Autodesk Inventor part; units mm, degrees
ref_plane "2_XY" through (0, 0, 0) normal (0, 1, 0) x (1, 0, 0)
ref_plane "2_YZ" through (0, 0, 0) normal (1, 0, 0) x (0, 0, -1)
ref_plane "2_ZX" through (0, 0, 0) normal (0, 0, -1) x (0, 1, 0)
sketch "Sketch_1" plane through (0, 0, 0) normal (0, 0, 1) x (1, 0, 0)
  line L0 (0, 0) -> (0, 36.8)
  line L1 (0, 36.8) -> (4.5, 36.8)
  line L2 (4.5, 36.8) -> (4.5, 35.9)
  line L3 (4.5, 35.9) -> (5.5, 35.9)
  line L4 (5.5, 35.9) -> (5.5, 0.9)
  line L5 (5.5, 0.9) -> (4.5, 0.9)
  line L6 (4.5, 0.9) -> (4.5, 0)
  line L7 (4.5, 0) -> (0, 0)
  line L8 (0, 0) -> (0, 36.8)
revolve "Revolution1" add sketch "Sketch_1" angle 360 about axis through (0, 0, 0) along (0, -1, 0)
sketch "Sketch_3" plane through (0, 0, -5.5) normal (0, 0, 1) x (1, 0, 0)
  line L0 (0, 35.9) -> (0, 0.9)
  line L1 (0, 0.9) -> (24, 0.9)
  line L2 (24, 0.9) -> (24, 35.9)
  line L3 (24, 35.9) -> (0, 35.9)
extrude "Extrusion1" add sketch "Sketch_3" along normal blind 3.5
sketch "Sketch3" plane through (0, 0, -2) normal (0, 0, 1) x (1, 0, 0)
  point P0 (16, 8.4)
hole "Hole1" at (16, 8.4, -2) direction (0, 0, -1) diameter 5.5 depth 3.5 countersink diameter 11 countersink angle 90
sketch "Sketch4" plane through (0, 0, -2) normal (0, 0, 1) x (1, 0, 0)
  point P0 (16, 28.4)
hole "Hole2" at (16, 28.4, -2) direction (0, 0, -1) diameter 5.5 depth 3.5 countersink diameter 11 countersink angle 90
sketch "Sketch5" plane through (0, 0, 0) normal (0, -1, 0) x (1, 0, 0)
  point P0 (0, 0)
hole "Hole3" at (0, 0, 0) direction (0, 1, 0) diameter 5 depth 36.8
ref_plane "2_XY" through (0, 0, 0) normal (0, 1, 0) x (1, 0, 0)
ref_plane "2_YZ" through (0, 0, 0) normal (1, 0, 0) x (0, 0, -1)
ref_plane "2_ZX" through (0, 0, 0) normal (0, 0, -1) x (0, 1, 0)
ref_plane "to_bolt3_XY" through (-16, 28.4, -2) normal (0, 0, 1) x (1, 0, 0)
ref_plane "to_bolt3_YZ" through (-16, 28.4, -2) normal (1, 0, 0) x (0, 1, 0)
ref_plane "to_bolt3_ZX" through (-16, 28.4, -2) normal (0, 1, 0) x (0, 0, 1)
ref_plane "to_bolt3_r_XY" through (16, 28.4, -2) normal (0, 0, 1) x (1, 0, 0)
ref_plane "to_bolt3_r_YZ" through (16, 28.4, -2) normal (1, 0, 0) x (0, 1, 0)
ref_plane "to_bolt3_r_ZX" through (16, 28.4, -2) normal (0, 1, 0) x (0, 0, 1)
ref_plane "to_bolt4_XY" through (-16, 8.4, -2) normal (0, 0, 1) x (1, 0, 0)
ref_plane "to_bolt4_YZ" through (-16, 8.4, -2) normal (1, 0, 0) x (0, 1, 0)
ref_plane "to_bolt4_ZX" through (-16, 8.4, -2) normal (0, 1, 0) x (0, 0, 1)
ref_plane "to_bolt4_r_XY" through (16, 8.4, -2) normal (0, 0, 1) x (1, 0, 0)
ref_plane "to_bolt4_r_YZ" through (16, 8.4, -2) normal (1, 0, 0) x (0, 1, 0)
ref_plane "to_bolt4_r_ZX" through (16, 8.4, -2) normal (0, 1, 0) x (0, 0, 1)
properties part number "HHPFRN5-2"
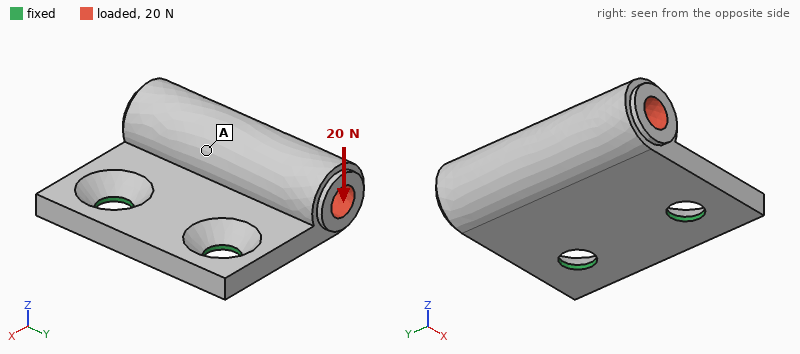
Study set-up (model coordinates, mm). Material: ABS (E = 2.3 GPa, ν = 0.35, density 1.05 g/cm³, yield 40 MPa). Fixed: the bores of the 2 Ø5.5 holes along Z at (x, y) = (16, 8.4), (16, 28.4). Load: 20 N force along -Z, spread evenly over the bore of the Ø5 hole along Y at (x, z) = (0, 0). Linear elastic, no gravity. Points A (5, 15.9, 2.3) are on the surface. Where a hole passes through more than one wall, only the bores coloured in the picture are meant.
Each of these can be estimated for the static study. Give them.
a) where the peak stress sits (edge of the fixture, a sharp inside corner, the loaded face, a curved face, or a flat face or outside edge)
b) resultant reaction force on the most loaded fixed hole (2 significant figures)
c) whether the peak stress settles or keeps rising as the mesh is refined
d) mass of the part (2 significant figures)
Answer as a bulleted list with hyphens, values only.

- edge of the fixture
- 11 N
- keeps rising
- 5.1 g
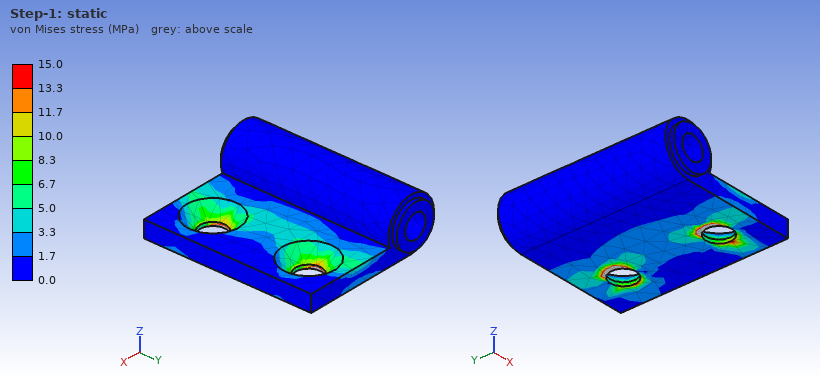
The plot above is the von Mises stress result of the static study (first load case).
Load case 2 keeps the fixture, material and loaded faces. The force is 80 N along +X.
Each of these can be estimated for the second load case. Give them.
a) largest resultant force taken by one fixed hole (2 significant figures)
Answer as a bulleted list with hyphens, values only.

- 40 N
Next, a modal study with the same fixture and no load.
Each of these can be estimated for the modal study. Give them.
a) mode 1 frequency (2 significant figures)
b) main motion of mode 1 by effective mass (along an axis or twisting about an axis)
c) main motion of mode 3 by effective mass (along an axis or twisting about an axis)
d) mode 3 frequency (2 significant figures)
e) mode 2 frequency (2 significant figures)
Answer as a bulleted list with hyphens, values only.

- 800 Hz
- along Z
- along Y
- 4600 Hz
- 2300 Hz
